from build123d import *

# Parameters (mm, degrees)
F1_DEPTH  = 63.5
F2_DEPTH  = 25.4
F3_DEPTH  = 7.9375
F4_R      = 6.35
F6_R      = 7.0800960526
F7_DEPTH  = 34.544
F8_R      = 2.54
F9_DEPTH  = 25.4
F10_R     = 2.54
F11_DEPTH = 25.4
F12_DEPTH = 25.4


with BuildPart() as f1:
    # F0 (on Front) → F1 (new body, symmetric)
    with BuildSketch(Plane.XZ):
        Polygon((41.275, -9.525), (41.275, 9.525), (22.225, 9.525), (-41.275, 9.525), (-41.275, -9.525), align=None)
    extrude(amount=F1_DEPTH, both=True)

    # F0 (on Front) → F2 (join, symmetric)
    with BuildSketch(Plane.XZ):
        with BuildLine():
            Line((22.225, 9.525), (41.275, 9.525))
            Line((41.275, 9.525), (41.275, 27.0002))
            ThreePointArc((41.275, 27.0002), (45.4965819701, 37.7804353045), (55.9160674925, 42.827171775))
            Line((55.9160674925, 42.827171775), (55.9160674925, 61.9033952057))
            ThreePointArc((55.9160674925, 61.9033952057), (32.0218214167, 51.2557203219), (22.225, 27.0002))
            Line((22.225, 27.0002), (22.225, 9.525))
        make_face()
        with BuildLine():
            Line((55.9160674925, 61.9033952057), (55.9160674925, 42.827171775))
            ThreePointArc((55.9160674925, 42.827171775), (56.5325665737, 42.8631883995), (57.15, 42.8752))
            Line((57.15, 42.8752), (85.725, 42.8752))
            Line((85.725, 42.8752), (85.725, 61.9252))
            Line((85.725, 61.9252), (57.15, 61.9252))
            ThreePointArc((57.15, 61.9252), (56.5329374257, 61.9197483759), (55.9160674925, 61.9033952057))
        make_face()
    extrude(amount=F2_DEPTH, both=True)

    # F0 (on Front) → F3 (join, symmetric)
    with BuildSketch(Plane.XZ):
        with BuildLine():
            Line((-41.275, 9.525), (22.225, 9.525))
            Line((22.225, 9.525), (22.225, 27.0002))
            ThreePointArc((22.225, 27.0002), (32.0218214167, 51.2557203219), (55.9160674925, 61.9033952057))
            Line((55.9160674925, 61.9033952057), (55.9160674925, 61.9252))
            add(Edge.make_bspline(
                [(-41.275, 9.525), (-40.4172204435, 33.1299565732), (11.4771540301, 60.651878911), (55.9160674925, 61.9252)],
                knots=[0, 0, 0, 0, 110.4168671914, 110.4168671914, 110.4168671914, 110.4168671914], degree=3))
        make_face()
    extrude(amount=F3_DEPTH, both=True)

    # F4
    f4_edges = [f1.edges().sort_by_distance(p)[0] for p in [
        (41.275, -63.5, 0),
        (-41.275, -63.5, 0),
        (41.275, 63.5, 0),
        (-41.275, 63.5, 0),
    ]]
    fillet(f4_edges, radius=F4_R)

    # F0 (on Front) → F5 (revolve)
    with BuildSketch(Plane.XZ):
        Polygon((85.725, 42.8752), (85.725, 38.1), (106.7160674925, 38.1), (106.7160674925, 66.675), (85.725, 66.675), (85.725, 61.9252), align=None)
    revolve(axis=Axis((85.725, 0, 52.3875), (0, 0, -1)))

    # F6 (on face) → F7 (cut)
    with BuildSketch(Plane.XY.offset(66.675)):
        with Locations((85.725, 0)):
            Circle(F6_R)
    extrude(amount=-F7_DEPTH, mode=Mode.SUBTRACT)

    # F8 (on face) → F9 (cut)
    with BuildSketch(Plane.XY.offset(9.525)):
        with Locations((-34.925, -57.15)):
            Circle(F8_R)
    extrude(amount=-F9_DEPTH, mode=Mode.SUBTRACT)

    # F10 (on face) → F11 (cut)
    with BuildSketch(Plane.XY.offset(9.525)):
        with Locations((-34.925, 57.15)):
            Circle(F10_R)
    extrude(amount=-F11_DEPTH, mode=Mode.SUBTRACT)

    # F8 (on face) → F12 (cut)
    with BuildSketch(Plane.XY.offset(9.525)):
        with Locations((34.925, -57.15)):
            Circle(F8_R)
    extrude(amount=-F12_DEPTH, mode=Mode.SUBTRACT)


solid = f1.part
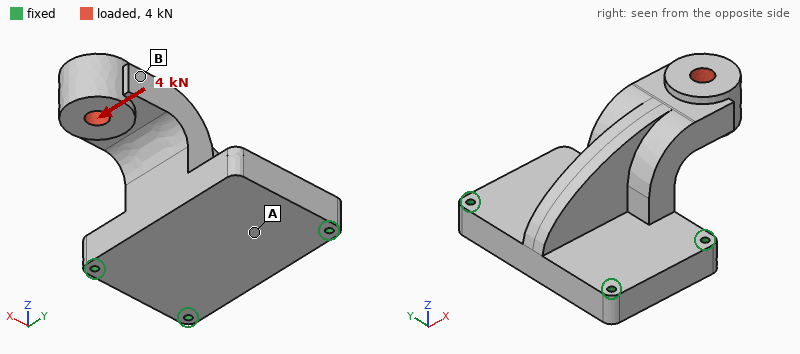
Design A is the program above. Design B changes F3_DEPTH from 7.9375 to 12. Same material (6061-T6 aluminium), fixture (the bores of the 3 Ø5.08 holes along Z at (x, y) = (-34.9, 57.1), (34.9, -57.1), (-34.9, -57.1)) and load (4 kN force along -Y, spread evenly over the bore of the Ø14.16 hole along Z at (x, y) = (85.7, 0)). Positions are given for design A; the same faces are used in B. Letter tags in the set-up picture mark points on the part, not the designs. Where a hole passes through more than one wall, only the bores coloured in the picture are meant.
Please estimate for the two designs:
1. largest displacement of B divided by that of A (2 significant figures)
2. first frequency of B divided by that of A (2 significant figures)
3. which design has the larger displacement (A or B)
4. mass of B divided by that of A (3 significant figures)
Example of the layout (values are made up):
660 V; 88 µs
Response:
0.86; 1.0; A; 1.05
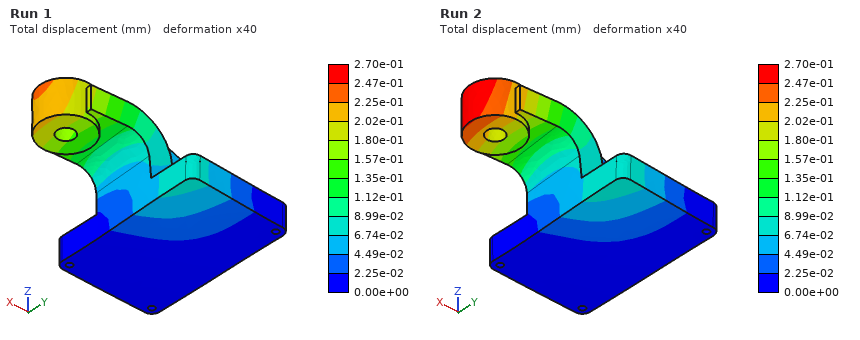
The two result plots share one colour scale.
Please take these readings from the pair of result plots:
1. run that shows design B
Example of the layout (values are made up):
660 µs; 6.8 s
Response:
Run 1
